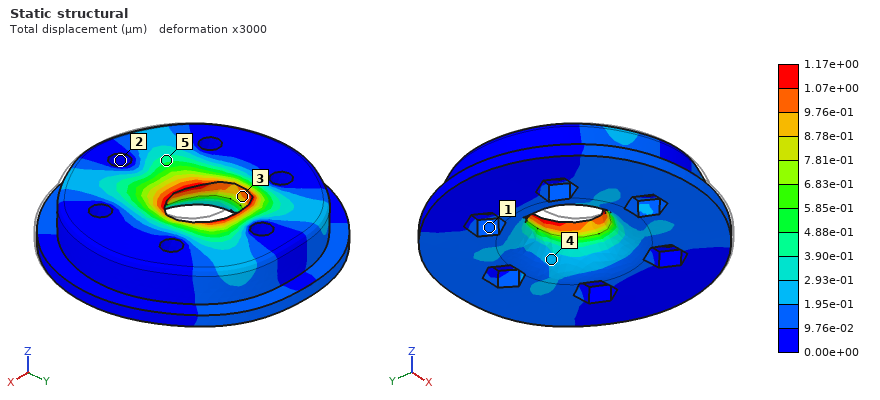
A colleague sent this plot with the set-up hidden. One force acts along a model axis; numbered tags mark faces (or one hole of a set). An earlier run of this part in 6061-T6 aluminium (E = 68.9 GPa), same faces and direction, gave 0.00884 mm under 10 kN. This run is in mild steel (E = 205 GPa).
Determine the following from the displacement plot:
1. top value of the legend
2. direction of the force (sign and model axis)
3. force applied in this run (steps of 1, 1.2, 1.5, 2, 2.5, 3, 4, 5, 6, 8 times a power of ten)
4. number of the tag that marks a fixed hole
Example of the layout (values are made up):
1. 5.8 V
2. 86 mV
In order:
1. 1.17e+00 µm
2. +Y
3. 4 kN
4. 2
